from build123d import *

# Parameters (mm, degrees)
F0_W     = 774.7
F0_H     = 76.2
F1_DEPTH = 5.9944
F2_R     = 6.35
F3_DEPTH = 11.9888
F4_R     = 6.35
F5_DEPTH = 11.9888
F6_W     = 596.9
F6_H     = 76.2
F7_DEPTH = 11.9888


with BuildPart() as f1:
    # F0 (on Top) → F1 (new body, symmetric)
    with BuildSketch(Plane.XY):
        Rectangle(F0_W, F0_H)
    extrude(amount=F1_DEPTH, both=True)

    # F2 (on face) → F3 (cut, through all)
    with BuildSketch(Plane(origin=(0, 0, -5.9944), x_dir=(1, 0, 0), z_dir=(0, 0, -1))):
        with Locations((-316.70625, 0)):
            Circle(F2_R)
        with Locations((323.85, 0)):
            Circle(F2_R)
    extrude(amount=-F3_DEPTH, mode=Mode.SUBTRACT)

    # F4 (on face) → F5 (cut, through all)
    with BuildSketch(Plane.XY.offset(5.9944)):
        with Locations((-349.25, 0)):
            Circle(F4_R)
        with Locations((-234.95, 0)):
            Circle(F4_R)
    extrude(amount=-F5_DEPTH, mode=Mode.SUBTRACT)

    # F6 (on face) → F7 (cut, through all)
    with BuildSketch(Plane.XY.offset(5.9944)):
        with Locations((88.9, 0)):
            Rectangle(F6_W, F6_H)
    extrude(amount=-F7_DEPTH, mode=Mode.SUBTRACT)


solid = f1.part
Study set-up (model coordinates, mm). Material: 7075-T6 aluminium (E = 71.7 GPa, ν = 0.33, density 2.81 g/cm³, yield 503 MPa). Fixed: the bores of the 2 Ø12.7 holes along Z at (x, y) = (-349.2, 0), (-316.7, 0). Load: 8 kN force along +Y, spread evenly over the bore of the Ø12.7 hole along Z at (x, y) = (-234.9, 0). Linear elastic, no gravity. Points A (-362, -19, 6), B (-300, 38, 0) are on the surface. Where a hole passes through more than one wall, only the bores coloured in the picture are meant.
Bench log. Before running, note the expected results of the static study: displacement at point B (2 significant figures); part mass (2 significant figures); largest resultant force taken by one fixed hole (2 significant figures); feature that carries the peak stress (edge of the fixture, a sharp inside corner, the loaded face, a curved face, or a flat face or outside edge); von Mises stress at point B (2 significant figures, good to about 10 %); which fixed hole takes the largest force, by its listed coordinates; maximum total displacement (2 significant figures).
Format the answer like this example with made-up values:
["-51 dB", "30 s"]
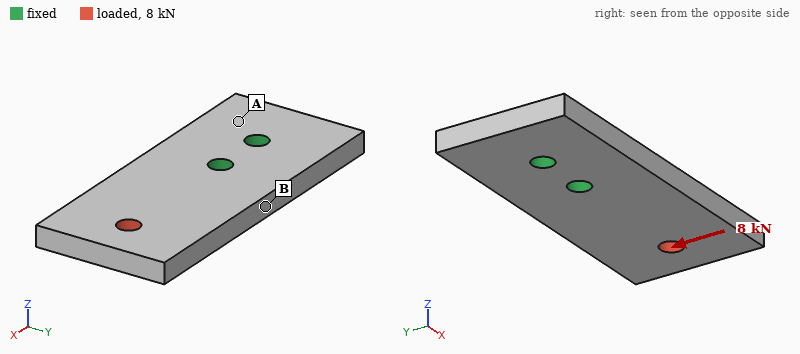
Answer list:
["0.057 mm", "440 g", "21 kN", "edge of the fixture", "50 MPa", "(-316.7, 0)", "0.21 mm"]
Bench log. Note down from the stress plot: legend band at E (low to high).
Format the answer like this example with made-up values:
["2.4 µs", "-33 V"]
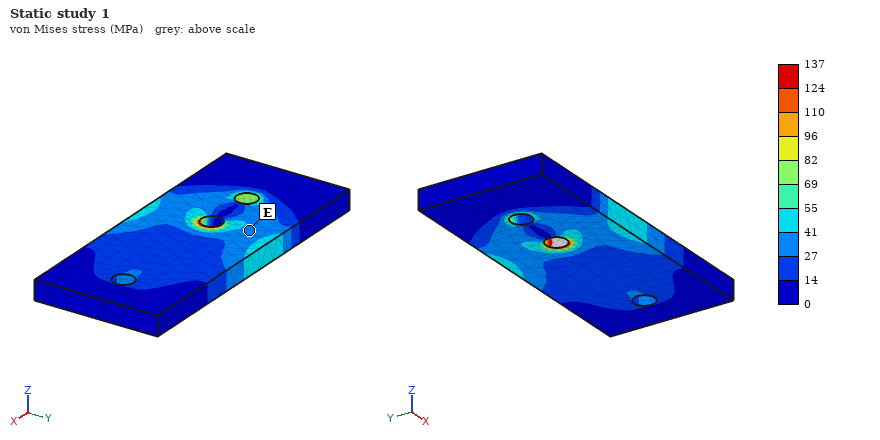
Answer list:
["27 to 41 MPa"]
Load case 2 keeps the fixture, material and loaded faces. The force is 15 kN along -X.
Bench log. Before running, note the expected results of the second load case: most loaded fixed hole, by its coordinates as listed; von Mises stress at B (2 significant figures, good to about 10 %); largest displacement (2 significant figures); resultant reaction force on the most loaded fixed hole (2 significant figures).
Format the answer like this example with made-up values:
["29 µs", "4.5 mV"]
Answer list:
["(-316.7, 0)", "9.8 MPa", "33 µm", "11 kN"]
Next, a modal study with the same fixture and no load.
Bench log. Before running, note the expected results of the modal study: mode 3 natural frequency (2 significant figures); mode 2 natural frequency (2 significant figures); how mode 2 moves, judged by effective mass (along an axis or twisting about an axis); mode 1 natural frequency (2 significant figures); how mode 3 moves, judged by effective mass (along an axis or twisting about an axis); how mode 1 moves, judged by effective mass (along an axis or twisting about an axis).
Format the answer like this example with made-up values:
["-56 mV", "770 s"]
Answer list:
["2800 Hz", "2200 Hz", "twisting about X", "860 Hz", "along Y", "along Z"]
